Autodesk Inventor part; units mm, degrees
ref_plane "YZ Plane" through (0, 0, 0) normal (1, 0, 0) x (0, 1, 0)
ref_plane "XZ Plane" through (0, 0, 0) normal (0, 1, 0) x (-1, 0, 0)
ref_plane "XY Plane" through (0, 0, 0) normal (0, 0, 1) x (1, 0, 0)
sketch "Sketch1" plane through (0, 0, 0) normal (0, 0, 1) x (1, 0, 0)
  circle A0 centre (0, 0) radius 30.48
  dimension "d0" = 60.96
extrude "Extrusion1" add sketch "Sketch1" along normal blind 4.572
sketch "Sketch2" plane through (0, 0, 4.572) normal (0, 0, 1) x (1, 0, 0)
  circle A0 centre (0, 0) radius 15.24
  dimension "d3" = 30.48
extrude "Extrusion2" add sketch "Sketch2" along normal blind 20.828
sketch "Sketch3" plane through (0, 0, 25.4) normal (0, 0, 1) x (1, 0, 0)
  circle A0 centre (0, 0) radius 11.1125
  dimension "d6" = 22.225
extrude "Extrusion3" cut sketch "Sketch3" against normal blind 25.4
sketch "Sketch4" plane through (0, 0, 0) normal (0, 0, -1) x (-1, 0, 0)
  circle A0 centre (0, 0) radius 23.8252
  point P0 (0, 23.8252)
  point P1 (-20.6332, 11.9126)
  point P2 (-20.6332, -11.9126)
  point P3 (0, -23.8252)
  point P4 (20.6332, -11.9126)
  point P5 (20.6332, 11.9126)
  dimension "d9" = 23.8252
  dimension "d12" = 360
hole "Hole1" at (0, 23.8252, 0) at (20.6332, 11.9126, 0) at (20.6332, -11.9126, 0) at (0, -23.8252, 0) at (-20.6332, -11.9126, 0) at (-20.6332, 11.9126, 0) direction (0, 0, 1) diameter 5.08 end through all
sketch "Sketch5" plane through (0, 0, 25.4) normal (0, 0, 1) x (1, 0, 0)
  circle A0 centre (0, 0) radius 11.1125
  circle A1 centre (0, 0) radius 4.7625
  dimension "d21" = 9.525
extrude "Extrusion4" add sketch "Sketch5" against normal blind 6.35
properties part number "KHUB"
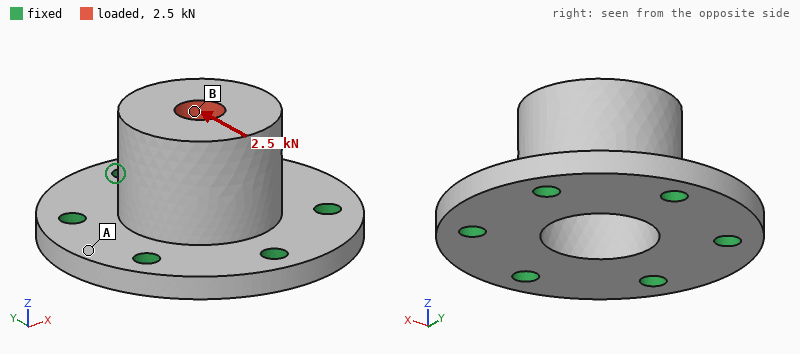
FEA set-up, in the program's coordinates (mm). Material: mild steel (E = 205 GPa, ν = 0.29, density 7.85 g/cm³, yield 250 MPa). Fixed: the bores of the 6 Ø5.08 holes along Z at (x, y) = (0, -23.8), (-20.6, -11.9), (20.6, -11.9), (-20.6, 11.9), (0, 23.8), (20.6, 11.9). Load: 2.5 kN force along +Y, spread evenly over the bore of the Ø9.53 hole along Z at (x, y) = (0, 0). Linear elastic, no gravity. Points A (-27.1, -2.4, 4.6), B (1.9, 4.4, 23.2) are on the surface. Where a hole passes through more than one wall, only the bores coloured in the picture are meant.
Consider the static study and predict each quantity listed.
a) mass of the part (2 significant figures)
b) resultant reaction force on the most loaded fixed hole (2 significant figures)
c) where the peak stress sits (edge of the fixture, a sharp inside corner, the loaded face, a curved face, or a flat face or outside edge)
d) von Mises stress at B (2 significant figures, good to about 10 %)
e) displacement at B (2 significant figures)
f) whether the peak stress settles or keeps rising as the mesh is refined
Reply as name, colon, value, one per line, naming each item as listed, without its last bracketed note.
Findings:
mass of the part: 160 g
resultant reaction force on the most loaded fixed hole: 1.1 kN
where the peak stress sits: edge of the fixture
von Mises stress at B: 16 MPa
displacement at B: 9.6 µm
whether the peak stress settles or keeps rising as the mesh is refined: keeps rising
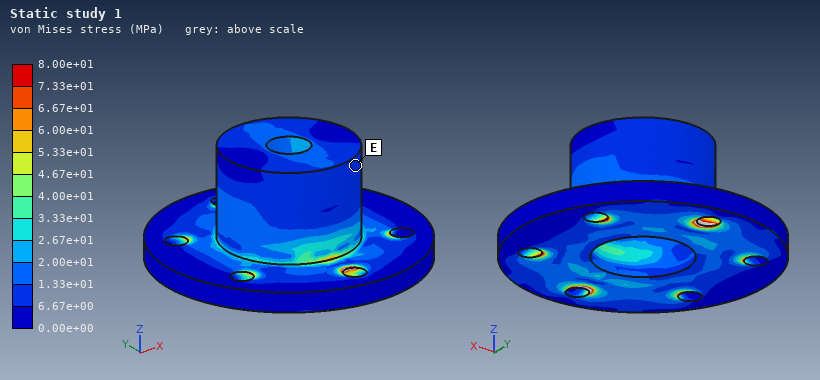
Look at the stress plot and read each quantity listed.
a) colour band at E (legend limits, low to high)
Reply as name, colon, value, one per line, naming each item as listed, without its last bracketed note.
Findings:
colour band at E: 6.67e+00 to 1.33e+01 MPa
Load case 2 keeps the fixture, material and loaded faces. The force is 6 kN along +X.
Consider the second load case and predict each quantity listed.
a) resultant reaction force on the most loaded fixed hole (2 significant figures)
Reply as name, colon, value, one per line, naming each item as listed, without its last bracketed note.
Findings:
resultant reaction force on the most loaded fixed hole: 2.2 kN
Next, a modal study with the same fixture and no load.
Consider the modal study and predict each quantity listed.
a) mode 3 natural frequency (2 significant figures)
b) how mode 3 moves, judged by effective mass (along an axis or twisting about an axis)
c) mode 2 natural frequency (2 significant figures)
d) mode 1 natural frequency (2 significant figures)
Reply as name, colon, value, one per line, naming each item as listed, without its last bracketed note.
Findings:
mode 3 natural frequency: 16 kHz
how mode 3 moves, judged by effective mass: along Z
mode 2 natural frequency: 12 kHz
mode 1 natural frequency: 12 kHz
